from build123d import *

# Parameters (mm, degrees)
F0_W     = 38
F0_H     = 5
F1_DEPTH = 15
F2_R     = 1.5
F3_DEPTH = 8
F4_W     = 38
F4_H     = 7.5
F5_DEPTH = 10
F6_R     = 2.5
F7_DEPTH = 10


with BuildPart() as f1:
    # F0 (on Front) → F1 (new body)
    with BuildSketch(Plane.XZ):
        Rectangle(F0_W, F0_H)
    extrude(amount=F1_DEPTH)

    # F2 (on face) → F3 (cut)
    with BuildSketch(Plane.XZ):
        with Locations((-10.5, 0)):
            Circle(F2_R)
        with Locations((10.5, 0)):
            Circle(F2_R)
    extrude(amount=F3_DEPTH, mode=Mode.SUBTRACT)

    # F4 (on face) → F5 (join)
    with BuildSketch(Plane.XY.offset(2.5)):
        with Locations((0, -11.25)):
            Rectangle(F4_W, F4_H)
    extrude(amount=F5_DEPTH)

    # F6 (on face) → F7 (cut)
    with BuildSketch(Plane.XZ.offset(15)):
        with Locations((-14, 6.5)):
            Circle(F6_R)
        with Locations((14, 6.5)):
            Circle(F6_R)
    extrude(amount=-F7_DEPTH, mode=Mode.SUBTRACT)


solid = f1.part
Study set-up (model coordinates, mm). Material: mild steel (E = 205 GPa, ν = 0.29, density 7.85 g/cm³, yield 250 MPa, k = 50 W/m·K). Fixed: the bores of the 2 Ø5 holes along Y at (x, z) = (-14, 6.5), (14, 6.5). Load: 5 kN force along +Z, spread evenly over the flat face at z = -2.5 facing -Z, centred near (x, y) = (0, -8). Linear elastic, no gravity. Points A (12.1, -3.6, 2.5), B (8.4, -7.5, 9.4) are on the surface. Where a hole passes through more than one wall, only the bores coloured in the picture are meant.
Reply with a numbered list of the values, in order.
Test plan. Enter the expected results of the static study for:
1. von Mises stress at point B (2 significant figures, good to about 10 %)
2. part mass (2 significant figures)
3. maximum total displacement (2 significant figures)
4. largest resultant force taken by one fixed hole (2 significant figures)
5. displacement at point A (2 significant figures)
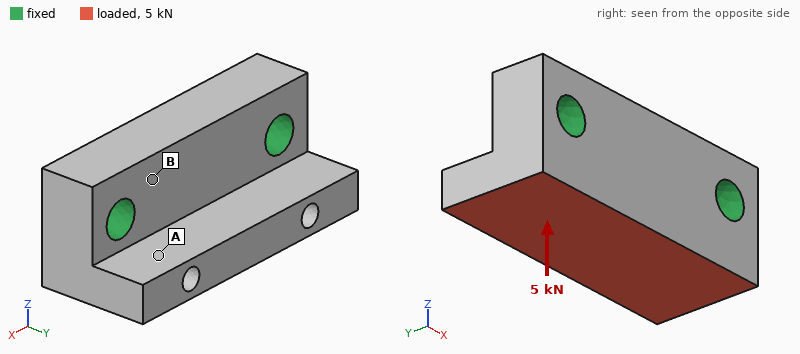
1. 43 MPa
2. 42 g
3. 13 µm
4. 2.5 kN
5. 6.6 µm
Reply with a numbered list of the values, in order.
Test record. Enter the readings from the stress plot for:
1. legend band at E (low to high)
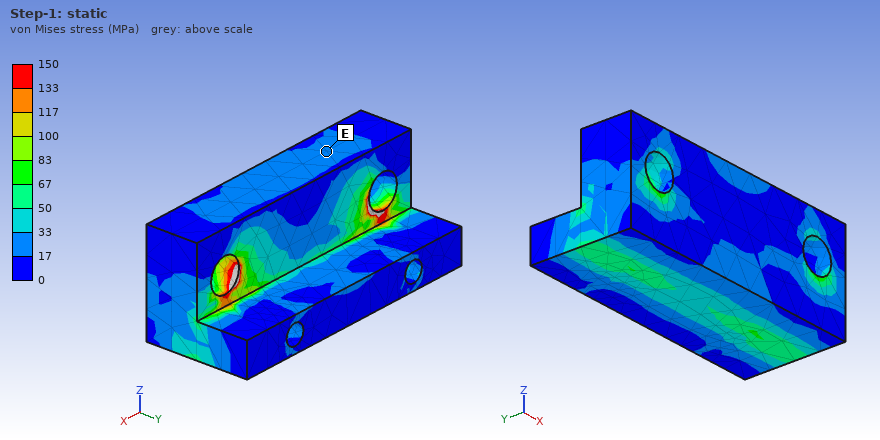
1. 17 to 33 MPa
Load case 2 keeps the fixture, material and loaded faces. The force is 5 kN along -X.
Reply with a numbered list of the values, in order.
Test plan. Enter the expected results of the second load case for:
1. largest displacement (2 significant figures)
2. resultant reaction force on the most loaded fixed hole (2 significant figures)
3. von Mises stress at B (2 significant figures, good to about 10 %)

1. 5.4 µm
2. 2.9 kN
3. 11 MPa
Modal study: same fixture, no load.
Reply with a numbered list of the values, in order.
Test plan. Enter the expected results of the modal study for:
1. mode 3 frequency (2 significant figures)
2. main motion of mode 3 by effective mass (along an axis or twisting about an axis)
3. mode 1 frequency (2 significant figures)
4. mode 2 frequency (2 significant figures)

1. 39 kHz
2. along Y
3. 24 kHz
4. 34 kHz
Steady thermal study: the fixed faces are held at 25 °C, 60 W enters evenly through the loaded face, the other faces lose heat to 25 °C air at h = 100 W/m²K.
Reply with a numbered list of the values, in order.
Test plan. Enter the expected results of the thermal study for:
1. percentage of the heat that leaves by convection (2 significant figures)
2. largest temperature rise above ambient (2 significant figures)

1. 7.6 %
2. 52 K
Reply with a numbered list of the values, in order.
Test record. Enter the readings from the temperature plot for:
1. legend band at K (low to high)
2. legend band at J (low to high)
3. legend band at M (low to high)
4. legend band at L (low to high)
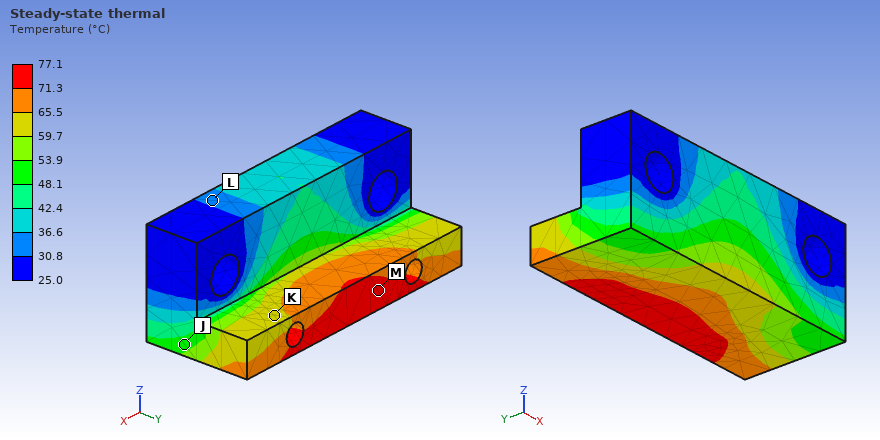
1. 59.7 to 65.5 °C
2. 48.1 to 53.9 °C
3. 71.3 to 77.1 °C
4. 30.8 to 36.6 °C
